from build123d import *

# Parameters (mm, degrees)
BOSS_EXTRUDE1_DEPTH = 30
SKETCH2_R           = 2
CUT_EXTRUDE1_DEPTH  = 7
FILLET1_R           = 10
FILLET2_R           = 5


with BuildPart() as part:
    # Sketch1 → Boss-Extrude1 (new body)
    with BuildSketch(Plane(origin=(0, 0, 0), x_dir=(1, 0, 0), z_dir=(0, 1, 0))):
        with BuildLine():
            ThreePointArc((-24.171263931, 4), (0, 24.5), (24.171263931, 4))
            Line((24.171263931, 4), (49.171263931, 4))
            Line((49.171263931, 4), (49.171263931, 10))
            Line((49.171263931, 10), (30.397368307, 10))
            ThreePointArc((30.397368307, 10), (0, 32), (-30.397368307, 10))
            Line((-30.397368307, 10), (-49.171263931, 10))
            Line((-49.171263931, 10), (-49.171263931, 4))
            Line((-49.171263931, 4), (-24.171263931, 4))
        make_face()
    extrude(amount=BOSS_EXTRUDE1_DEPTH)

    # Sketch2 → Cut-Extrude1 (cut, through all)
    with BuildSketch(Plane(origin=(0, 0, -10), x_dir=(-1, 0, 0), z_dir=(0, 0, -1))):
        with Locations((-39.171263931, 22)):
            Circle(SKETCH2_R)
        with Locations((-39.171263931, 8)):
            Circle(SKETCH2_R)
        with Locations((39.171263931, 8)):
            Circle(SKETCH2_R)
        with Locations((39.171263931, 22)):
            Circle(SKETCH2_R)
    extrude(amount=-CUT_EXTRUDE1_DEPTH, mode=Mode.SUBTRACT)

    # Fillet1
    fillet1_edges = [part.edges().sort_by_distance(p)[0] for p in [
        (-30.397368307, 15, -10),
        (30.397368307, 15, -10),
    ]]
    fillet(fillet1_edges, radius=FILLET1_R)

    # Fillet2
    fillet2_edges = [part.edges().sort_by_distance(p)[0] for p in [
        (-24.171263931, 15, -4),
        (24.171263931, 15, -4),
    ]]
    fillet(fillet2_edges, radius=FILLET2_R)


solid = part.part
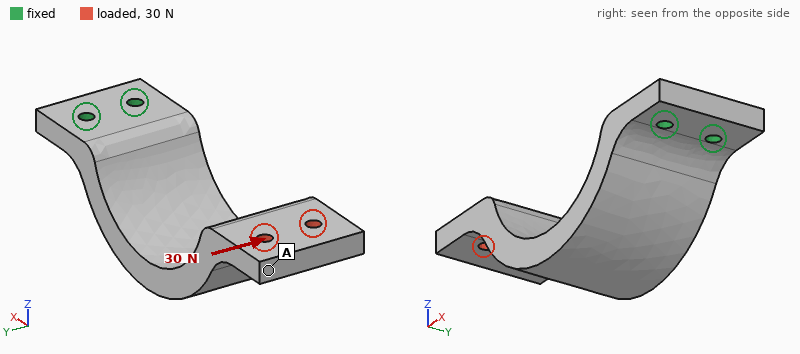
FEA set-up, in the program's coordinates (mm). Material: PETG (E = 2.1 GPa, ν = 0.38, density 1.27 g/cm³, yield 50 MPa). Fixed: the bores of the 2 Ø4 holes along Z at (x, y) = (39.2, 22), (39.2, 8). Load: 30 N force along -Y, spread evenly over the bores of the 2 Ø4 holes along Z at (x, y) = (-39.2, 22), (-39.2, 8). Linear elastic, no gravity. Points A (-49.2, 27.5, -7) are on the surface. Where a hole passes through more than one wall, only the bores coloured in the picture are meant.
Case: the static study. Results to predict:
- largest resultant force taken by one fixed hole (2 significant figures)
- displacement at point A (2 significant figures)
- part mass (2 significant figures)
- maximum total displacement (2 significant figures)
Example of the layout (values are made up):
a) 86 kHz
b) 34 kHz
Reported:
a) 140 N
b) 1.0 mm
c) 31 g
d) 1.1 mm
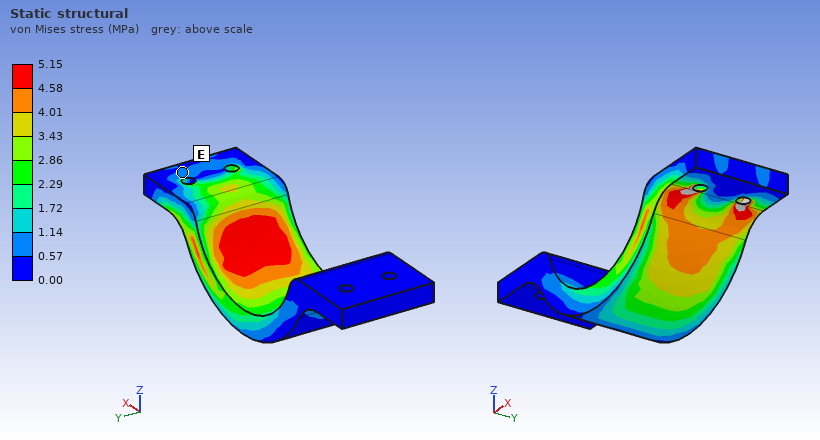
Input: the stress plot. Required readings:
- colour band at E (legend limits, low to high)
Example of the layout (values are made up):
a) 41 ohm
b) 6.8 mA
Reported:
a) 0.57 to 1.14 MPa
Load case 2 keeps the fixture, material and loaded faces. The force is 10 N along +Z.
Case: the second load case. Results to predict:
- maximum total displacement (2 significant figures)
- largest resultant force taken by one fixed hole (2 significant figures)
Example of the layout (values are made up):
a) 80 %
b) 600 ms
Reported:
a) 1.1 mm
b) 6.4 N
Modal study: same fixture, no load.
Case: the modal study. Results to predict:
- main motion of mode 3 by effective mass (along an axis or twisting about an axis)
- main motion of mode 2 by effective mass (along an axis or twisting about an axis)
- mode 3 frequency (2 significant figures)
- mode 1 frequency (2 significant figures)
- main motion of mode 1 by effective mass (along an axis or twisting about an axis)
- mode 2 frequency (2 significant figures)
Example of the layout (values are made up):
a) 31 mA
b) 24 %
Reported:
a) along X
b) along Y
c) 610 Hz
d) 170 Hz
e) along Z
f) 320 Hz
